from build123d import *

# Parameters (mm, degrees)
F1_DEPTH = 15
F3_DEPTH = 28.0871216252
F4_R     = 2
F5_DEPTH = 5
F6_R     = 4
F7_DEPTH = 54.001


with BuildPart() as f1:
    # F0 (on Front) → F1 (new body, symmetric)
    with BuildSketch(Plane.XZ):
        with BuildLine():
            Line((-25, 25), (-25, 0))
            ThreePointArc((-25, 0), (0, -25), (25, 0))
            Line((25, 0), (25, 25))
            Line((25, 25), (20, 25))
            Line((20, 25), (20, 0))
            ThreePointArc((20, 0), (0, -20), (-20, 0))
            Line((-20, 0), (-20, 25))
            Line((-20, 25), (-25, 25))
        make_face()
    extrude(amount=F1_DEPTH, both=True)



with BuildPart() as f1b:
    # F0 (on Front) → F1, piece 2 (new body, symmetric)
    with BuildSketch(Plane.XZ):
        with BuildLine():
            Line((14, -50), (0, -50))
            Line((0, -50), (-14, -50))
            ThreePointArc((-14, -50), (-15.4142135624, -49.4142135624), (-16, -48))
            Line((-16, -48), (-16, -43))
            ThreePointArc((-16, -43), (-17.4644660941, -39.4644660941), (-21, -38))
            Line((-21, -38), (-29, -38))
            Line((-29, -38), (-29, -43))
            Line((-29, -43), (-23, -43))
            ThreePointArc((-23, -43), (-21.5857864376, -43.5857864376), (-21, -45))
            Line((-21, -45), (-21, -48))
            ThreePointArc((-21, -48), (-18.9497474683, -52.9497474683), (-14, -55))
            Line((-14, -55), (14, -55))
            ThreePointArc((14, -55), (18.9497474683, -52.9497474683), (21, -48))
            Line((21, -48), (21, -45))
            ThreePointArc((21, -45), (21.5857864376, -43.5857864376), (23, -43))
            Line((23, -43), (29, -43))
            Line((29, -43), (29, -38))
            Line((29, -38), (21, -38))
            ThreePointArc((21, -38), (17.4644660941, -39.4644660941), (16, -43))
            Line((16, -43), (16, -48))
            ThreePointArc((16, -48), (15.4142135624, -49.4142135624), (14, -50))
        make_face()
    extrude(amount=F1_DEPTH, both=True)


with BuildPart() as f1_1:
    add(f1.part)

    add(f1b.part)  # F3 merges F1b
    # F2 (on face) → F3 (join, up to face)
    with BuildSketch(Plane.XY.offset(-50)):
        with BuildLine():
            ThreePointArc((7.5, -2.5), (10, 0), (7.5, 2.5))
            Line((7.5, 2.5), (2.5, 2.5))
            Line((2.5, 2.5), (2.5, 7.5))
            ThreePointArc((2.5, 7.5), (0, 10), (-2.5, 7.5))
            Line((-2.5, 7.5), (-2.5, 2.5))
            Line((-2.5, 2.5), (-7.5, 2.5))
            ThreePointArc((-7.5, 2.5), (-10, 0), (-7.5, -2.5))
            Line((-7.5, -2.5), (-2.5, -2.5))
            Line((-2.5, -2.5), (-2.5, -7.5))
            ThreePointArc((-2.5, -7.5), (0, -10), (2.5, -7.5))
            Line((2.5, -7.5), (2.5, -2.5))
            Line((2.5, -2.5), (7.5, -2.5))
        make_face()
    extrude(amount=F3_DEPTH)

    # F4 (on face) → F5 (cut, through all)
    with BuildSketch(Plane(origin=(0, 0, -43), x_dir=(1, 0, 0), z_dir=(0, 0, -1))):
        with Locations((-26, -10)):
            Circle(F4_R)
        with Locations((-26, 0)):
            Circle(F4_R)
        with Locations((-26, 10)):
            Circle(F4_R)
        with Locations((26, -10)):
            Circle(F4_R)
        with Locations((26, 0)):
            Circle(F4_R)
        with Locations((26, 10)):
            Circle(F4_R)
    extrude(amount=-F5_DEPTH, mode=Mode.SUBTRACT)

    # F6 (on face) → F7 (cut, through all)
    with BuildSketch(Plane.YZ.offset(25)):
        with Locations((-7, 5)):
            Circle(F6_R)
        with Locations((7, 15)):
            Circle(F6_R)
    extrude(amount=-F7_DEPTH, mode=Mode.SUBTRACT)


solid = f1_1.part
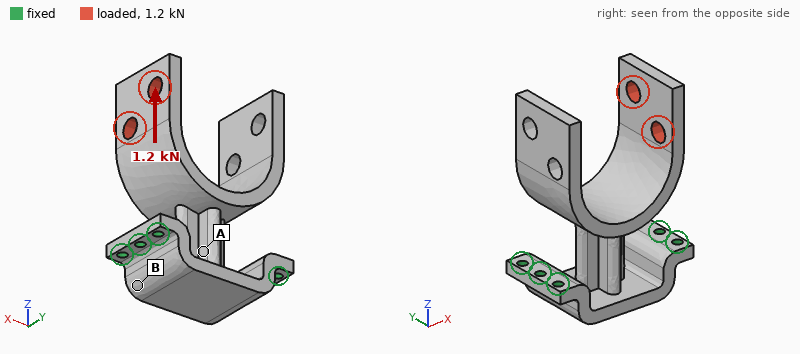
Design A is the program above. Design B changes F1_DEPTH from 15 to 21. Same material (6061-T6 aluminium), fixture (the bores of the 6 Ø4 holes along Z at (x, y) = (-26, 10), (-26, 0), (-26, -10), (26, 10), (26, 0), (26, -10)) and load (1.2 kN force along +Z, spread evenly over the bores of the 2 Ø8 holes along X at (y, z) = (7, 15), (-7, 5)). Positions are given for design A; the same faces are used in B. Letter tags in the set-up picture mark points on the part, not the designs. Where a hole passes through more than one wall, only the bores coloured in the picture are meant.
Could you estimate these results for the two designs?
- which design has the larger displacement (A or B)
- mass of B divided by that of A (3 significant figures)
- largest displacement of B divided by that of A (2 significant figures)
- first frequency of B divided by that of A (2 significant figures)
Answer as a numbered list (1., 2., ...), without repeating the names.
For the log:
1. A
2. 1.37
3. 0.86
4. 0.88
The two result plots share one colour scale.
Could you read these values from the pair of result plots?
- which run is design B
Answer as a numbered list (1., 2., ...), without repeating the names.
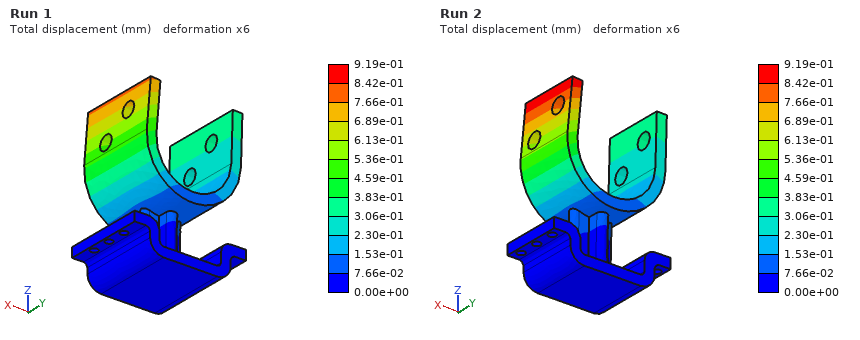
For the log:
1. Run 1
